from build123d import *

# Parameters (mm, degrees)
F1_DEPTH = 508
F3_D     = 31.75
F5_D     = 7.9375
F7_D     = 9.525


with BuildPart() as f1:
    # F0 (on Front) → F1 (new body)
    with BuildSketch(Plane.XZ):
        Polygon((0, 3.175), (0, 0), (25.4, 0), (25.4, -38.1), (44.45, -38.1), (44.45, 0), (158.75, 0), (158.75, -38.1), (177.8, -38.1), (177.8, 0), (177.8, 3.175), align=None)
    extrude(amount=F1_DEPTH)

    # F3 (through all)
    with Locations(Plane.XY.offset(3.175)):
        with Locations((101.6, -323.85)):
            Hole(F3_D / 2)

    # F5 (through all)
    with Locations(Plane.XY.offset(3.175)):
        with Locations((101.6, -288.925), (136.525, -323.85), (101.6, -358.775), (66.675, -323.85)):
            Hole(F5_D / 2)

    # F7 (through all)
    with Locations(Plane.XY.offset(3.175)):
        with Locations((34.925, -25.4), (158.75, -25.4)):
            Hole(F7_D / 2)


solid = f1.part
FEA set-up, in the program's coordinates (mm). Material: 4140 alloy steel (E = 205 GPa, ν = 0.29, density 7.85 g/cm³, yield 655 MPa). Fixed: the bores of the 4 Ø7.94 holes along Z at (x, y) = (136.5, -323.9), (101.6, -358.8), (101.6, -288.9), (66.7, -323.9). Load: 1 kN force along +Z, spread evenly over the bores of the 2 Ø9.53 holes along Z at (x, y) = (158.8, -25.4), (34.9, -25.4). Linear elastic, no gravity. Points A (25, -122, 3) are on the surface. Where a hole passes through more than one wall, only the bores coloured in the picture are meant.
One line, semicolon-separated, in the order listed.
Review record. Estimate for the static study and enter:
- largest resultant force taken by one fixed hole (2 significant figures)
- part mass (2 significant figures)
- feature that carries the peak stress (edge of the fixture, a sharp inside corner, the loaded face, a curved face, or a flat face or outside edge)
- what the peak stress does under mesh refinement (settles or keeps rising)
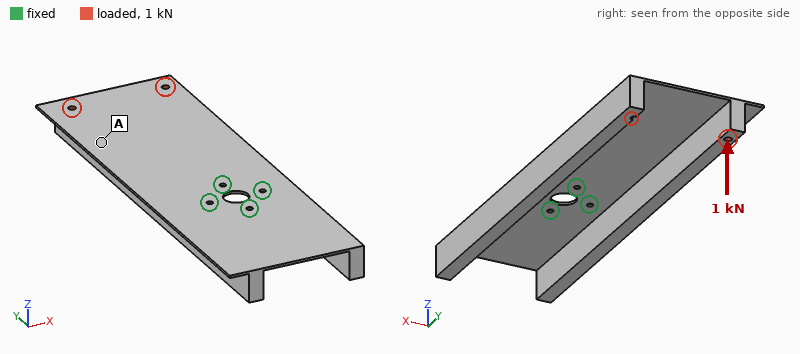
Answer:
2.5 kN; 8.0 kg; edge of the fixture; keeps rising
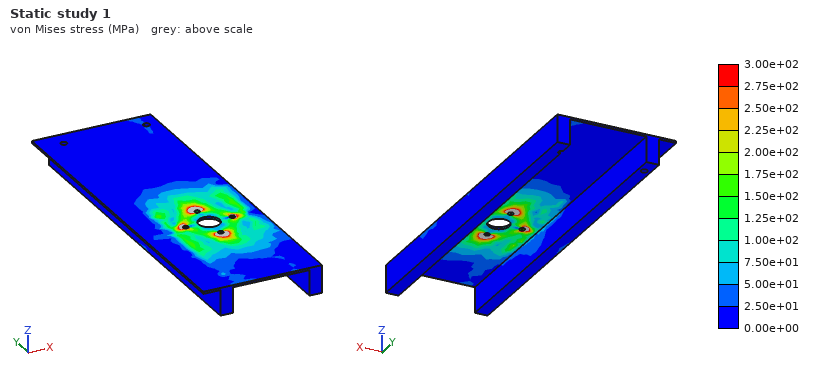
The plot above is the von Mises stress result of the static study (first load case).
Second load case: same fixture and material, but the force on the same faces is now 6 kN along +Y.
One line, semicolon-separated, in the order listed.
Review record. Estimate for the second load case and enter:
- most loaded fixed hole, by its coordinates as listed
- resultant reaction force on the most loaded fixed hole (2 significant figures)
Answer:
(66.7, -323.9); 3.0 kN
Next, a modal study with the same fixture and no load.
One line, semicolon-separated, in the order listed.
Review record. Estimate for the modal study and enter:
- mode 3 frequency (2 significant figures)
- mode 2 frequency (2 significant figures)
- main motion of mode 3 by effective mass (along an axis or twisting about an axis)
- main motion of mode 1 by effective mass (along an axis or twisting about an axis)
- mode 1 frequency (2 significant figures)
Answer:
220 Hz; 140 Hz; along Z; along Z; 58 Hz
